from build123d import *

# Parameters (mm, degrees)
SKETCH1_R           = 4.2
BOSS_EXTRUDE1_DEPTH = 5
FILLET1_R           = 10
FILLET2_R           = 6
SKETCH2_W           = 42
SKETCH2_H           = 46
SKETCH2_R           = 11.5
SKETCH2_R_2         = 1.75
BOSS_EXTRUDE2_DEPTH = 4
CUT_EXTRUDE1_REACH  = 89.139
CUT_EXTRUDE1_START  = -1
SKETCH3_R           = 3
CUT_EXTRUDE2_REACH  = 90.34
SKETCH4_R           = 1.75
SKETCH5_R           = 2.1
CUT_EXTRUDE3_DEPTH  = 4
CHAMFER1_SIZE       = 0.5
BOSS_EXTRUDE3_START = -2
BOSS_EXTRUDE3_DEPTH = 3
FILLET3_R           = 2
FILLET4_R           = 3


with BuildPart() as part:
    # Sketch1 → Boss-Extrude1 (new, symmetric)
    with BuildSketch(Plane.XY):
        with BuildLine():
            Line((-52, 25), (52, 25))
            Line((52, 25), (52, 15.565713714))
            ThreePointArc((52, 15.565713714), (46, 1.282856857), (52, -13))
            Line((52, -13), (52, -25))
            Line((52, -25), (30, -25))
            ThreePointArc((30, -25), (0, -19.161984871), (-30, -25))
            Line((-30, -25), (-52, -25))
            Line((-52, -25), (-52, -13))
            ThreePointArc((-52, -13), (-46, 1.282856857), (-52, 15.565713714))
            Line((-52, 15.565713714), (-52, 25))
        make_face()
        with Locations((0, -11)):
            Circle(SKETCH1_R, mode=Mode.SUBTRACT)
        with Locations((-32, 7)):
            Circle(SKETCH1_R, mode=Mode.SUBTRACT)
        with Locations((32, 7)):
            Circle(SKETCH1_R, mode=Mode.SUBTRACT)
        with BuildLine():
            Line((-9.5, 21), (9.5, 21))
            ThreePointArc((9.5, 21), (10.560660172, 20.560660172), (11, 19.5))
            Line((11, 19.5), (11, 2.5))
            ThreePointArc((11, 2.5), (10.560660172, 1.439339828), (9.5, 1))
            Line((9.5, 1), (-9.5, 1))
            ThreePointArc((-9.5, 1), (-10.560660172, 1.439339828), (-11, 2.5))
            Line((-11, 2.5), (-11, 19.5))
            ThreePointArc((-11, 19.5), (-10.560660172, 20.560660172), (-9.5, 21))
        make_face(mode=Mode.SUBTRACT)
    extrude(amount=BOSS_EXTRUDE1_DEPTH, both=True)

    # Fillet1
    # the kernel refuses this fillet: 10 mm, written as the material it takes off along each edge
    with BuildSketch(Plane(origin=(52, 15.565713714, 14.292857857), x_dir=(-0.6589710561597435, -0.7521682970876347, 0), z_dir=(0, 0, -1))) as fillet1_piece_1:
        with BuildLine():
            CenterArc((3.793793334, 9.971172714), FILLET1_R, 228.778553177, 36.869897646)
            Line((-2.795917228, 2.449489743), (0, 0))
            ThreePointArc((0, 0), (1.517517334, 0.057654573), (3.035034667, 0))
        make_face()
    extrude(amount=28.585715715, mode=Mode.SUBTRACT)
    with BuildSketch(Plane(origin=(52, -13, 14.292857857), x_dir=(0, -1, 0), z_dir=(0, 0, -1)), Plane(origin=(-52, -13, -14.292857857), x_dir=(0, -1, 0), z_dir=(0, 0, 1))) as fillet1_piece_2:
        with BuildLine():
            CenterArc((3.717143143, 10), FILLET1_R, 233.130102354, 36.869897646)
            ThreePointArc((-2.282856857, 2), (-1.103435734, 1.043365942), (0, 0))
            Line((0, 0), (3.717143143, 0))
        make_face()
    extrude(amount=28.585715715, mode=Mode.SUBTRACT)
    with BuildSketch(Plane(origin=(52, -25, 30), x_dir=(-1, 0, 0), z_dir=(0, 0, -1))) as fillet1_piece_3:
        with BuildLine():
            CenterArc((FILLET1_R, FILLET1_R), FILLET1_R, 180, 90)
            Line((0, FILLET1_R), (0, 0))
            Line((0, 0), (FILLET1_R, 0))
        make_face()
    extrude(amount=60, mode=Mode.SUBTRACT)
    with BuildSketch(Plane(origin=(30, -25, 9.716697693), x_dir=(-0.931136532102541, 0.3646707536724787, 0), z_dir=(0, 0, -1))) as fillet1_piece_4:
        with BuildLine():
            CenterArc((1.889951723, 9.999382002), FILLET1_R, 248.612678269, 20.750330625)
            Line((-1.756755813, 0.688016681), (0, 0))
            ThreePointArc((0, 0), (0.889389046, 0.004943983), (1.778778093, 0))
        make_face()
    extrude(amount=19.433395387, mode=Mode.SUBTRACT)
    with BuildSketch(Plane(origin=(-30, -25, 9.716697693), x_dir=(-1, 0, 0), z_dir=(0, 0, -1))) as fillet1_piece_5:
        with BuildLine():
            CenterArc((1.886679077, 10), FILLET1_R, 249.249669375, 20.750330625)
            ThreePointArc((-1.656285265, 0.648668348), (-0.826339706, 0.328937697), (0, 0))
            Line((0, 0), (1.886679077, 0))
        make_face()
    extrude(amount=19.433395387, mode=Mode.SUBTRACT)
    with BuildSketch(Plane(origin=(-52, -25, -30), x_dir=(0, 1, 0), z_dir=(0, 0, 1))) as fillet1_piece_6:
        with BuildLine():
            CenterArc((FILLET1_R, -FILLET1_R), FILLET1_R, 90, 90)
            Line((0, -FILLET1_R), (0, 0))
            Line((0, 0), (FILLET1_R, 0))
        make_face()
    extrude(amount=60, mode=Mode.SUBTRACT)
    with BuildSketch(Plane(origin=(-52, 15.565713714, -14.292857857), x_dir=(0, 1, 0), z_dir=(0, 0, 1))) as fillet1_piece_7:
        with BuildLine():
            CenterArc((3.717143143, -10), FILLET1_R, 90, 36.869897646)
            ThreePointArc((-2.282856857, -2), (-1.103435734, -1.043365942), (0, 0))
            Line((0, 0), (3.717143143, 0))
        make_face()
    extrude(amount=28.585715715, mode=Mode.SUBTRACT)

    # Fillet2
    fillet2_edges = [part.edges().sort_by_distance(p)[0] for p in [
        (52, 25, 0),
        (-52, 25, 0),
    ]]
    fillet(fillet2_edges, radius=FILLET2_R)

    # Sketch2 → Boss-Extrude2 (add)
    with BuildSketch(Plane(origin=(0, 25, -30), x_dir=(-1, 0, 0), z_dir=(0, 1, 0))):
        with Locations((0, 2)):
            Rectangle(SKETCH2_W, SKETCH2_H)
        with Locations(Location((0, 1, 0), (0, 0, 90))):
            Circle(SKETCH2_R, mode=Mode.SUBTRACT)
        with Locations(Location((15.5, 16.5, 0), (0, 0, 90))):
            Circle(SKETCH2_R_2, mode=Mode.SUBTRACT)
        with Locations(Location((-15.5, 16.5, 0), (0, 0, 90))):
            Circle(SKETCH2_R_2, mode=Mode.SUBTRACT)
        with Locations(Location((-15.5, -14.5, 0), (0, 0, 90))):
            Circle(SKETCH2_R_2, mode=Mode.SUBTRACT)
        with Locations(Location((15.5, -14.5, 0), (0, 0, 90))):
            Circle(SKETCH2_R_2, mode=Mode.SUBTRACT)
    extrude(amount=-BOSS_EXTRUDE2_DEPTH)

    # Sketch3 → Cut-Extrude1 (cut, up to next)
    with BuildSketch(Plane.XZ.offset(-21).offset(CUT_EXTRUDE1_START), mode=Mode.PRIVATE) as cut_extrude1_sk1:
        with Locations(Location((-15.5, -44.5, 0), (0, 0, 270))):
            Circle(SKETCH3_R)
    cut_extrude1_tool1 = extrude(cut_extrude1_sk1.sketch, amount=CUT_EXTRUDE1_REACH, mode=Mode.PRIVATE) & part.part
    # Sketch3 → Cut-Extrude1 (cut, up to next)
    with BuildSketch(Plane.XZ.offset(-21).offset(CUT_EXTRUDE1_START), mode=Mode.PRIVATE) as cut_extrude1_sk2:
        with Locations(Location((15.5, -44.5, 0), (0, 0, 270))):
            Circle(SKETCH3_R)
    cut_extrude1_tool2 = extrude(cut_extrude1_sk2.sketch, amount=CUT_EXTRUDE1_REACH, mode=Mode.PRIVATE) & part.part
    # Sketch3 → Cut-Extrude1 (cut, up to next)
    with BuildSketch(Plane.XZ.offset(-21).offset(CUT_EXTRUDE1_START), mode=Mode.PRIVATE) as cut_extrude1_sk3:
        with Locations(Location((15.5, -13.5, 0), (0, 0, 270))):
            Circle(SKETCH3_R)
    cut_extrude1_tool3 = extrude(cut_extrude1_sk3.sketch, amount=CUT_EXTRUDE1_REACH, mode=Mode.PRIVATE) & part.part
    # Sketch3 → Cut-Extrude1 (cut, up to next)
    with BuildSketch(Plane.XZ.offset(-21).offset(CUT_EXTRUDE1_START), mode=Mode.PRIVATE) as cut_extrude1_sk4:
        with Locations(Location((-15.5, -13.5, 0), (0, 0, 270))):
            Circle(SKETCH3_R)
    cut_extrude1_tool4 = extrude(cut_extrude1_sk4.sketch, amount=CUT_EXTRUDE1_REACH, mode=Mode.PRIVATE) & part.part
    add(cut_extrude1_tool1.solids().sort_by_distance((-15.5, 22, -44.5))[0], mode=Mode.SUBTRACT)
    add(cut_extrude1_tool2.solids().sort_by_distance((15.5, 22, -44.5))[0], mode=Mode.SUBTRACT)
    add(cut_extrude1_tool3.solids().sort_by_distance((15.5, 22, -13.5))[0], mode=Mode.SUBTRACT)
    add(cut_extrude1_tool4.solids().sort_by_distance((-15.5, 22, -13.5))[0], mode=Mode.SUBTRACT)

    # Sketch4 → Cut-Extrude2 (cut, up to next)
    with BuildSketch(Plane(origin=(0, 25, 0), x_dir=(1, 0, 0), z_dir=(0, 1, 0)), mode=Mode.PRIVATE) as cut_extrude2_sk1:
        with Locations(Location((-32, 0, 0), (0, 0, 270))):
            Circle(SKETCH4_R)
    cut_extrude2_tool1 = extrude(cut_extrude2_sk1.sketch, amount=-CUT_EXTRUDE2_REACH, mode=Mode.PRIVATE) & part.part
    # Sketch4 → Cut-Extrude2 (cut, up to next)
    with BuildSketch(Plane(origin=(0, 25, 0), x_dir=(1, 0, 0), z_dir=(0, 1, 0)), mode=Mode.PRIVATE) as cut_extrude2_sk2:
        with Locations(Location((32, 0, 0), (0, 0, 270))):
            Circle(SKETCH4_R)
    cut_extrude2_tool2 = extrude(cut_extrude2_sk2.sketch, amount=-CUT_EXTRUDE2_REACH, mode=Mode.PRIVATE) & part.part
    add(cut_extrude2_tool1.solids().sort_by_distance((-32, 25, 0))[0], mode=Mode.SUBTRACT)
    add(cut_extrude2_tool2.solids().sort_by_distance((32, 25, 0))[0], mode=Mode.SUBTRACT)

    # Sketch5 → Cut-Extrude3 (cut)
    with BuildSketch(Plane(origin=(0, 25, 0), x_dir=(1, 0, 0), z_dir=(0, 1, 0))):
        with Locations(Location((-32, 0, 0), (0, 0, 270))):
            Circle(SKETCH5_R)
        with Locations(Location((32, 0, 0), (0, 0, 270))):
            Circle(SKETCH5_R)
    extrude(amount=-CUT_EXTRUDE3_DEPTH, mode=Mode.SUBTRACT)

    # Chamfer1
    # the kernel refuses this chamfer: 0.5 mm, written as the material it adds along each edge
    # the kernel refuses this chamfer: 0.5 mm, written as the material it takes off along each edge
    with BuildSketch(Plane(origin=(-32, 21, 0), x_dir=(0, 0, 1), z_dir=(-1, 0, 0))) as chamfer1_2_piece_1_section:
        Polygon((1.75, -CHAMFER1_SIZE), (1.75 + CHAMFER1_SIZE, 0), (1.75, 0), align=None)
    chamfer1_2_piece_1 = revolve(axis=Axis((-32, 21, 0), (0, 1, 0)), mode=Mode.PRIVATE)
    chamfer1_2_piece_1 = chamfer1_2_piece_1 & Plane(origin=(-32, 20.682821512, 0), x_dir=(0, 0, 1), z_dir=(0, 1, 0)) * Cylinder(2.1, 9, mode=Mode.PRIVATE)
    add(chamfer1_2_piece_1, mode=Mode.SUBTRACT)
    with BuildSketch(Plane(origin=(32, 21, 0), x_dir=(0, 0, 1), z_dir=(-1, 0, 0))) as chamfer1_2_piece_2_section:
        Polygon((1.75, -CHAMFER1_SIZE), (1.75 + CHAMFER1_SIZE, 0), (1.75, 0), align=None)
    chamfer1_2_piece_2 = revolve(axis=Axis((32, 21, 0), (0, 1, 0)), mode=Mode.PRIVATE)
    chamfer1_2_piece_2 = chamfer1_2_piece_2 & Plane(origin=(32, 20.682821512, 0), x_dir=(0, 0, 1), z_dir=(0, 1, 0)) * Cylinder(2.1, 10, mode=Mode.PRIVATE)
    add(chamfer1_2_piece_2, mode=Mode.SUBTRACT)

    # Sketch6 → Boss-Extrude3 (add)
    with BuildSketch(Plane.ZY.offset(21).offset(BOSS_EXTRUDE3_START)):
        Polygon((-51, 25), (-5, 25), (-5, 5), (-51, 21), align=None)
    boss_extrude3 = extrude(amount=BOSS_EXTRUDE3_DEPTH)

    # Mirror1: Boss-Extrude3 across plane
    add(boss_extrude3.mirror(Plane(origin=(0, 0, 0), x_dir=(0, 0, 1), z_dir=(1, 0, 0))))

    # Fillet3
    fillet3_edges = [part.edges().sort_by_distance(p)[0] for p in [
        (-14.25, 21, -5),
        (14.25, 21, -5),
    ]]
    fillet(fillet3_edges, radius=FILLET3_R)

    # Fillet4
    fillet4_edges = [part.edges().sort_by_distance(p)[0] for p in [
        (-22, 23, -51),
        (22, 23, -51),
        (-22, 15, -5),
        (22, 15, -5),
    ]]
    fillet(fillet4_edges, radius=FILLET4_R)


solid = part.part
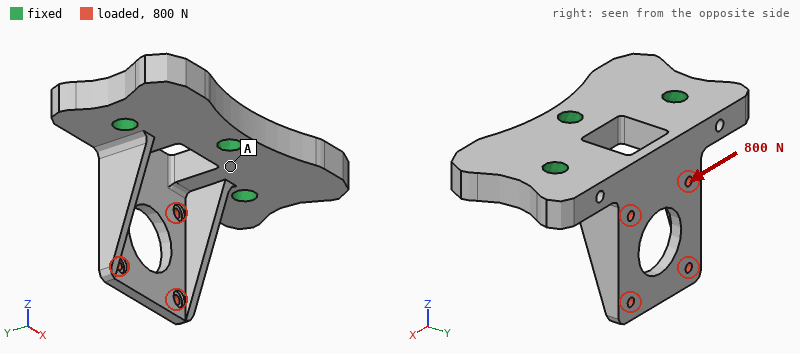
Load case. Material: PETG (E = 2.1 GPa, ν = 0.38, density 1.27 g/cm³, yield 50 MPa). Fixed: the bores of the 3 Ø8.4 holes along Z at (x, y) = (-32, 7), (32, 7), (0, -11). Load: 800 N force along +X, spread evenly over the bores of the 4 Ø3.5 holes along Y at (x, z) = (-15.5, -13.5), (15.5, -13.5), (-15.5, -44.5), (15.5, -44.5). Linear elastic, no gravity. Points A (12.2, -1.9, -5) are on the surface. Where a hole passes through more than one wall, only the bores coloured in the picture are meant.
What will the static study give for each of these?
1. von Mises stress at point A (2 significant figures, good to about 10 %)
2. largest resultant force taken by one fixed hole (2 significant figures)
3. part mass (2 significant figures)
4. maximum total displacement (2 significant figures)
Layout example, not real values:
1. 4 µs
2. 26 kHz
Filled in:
1. 3.4 MPa
2. 640 N
3. 62 g
4. 1.3 mm
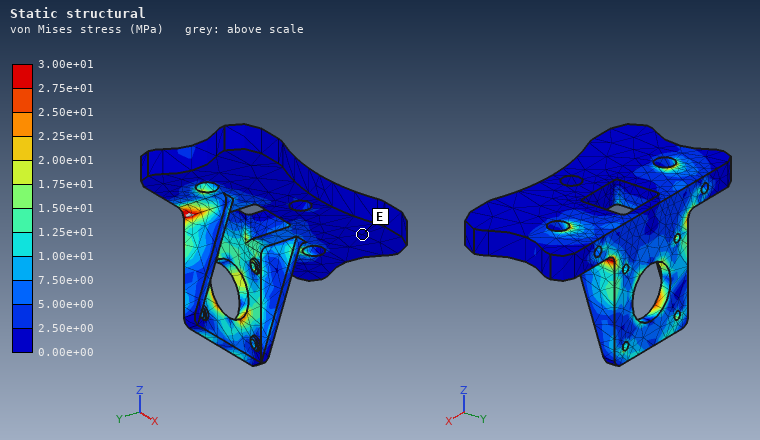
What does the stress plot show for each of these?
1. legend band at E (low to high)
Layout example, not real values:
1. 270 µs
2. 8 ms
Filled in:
1. 0.00e+00 to 2.50e+00 MPa
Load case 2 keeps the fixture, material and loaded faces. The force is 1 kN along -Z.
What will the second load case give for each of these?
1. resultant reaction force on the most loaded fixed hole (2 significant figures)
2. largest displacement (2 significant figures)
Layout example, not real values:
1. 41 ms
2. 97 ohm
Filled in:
1. 540 N
2. 1.4 mm
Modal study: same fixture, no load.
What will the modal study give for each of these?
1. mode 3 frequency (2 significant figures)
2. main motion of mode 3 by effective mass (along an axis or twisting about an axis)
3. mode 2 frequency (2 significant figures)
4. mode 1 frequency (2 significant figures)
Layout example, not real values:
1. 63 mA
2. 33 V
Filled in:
1. 2300 Hz
2. twisting about X
3. 1300 Hz
4. 920 Hz
